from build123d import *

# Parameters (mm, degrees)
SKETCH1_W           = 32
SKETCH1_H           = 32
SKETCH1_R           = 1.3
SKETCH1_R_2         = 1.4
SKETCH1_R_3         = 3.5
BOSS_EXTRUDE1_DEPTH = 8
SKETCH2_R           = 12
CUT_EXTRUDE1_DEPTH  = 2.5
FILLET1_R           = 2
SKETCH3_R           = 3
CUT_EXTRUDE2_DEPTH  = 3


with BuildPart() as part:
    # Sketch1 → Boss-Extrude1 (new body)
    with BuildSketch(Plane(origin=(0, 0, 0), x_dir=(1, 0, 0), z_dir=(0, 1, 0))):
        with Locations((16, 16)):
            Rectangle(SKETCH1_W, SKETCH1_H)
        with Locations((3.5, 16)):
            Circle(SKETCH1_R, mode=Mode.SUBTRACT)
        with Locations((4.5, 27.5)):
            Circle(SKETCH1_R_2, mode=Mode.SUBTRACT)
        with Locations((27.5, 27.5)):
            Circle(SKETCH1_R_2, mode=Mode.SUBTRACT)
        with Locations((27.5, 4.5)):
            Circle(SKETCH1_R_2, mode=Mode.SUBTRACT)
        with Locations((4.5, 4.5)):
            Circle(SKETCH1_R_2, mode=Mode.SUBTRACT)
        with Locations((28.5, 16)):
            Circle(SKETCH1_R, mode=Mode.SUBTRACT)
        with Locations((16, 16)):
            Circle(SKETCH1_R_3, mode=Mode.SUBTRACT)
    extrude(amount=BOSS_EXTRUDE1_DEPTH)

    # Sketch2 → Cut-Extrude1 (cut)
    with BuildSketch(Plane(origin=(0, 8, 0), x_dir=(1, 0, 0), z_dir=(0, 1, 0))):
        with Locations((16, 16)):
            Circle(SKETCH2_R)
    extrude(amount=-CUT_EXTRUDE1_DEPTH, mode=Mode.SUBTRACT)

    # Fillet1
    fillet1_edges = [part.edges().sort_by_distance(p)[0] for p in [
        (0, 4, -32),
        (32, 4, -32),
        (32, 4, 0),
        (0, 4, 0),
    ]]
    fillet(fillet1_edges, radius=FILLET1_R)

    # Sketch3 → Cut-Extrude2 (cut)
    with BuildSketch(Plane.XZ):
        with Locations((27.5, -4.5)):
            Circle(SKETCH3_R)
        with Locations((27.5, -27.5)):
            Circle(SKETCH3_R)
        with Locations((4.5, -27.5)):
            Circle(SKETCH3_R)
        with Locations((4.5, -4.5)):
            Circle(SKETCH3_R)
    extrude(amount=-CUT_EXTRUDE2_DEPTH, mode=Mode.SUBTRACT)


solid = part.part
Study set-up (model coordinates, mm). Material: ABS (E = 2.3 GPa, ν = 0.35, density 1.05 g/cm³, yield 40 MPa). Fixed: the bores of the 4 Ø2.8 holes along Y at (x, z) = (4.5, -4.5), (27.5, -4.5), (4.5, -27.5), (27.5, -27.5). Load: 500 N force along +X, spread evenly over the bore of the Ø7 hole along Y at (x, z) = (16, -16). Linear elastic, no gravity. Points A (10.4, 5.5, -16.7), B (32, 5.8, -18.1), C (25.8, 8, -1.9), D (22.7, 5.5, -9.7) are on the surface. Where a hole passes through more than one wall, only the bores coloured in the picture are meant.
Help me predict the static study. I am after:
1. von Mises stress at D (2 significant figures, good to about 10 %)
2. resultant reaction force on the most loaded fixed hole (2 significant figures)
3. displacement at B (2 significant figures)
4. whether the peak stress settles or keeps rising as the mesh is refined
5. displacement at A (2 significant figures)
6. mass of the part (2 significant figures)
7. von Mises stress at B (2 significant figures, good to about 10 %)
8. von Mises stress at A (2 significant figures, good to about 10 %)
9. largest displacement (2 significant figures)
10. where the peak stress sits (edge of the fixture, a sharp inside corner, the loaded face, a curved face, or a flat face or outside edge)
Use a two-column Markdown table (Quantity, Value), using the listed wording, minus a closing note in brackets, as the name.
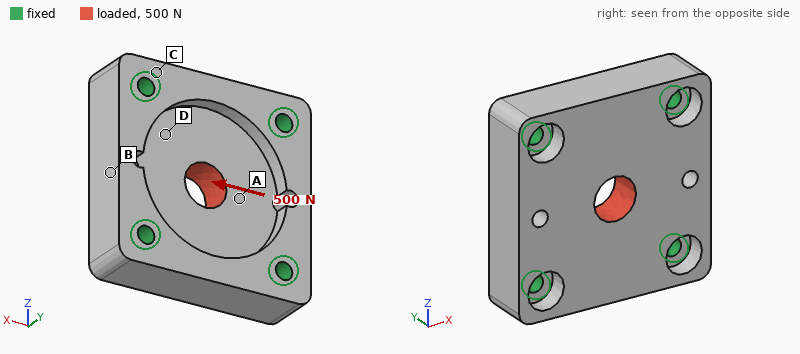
| Quantity | Value |
|---|---|
| von Mises stress at D | 4.0 MPa |
| resultant reaction force on the most loaded fixed hole | 130 N |
| displacement at B | 14 µm |
| whether the peak stress settles or keeps rising as the mesh is refined | keeps rising |
| displacement at A | 24 µm |
| mass of the part | 6.6 g |
| von Mises stress at B | 2.1 MPa |
| von Mises stress at A | 3.4 MPa |
| largest displacement | 29 µm |
| where the peak stress sits | edge of the fixture |
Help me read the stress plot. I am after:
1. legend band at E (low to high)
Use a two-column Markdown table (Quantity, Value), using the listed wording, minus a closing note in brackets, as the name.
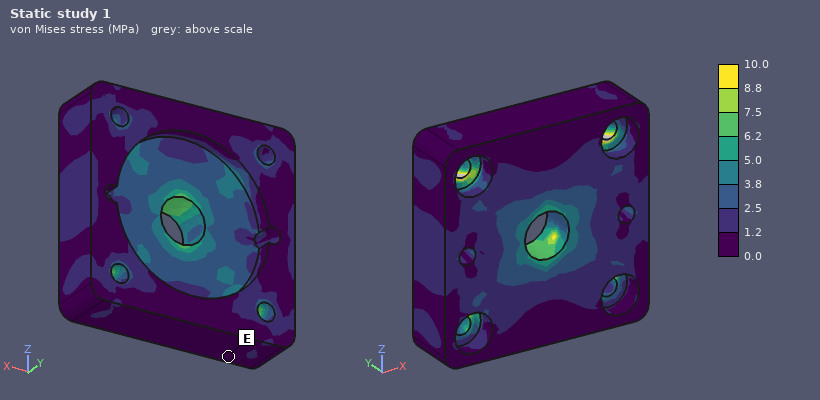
| Quantity | Value |
|---|---|
| legend band at E | 0.0 to 1.2 MPa |
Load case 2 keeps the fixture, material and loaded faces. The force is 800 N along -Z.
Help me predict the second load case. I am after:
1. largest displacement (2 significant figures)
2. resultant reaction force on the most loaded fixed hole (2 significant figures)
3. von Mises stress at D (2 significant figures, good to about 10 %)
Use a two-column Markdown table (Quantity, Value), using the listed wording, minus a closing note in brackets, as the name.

| Quantity | Value |
|---|---|
| largest displacement | 47 µm |
| resultant reaction force on the most loaded fixed hole | 210 N |
| von Mises stress at D | 6.4 MPa |
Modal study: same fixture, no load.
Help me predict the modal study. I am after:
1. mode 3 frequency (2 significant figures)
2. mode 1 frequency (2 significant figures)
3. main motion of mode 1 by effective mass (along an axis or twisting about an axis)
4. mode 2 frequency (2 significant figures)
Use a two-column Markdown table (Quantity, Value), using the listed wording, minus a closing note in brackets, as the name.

| Quantity | Value |
|---|---|
| mode 3 frequency | 13 kHz |
| mode 1 frequency | 9600 Hz |
| main motion of mode 1 by effective mass | along Y |
| mode 2 frequency | 13 kHz |
